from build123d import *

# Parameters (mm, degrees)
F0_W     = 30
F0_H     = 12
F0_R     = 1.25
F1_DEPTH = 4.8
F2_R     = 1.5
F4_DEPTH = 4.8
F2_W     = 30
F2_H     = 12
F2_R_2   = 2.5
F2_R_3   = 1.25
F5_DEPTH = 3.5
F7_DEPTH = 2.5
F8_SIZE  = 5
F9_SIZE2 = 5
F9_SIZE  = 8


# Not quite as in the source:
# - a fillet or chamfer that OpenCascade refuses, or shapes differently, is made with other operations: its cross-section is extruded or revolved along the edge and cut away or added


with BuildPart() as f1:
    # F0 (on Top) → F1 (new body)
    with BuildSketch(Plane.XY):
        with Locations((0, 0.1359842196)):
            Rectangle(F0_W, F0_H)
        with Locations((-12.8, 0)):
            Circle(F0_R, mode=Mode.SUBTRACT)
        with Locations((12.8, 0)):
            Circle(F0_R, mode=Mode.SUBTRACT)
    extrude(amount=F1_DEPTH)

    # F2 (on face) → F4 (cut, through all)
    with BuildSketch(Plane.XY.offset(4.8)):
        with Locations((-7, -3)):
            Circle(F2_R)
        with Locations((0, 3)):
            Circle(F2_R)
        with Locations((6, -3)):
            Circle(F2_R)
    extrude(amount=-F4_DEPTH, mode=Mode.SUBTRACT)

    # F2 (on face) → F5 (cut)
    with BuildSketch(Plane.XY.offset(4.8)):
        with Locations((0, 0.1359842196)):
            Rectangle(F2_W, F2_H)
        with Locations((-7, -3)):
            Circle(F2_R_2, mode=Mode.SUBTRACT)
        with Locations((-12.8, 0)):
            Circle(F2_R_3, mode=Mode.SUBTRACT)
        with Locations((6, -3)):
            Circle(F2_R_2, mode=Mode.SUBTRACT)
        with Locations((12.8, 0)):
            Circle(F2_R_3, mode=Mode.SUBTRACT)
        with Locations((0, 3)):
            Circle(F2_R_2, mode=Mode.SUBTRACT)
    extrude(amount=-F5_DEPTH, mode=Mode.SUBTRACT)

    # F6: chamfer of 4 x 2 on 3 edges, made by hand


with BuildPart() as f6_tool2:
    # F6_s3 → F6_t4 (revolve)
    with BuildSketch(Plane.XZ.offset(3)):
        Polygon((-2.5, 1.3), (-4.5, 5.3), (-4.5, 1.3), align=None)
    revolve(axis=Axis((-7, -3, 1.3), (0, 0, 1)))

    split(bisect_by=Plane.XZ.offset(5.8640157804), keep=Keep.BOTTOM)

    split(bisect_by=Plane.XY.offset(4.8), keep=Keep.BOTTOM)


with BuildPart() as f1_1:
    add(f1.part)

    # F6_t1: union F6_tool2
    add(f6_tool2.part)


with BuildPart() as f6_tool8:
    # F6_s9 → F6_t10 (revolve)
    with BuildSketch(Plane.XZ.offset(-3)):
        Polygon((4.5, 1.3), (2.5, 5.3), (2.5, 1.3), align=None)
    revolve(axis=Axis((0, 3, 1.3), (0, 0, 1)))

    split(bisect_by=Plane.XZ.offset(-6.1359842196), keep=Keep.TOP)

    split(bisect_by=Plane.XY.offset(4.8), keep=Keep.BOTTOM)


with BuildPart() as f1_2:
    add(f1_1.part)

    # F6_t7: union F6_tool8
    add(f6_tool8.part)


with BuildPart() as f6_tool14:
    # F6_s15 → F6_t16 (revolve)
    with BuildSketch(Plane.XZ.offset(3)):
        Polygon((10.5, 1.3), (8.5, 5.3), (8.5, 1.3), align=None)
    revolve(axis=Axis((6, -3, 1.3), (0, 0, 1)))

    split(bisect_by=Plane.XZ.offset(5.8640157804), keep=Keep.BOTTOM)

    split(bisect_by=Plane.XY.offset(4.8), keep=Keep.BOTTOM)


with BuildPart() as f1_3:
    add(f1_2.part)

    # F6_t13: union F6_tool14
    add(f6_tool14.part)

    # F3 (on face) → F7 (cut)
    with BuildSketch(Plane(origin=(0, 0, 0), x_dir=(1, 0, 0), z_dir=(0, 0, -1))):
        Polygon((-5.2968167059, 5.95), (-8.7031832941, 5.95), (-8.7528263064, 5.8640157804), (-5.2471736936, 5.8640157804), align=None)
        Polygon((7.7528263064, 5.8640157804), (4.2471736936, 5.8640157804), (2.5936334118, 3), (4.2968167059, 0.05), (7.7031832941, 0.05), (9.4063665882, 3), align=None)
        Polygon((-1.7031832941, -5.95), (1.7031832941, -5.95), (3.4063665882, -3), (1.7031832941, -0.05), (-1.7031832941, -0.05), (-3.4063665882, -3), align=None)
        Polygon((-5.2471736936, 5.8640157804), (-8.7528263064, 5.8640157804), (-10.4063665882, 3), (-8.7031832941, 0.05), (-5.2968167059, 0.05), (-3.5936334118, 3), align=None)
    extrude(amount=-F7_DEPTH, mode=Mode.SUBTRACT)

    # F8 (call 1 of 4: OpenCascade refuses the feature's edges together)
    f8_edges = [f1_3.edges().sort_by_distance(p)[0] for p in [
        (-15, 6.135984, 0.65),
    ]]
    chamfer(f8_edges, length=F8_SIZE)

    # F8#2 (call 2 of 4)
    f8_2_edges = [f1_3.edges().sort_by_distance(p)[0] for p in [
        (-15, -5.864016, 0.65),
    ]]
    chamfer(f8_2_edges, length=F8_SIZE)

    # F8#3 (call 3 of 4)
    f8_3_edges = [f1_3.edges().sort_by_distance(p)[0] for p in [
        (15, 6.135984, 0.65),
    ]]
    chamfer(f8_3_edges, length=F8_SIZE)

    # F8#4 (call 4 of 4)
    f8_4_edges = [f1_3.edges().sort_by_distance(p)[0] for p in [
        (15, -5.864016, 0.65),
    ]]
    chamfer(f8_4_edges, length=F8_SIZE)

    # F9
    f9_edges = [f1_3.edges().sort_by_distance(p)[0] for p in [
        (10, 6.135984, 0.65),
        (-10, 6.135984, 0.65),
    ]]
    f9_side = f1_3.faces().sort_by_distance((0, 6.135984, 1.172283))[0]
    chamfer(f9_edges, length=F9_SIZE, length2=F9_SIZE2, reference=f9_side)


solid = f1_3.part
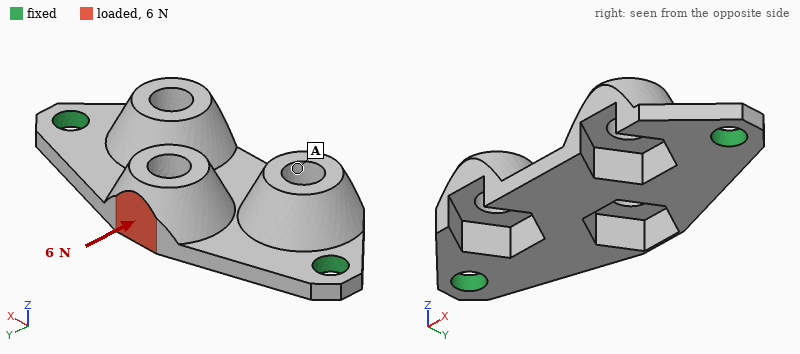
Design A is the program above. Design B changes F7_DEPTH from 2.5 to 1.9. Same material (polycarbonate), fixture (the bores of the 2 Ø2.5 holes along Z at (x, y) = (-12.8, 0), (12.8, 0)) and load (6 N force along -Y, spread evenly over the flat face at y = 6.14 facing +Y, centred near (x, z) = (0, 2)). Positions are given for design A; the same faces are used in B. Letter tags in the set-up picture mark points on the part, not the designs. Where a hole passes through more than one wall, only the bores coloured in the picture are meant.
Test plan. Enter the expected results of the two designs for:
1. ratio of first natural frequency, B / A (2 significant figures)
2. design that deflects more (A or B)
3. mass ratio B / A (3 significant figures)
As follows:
0.98
A
1.08
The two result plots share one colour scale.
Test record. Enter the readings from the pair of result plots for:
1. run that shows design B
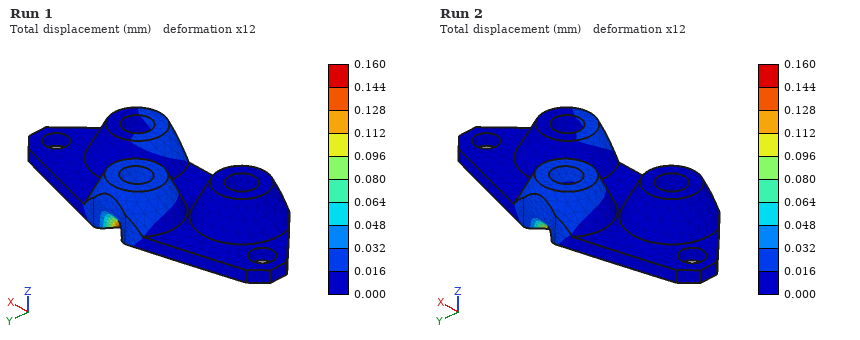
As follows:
Run 2
